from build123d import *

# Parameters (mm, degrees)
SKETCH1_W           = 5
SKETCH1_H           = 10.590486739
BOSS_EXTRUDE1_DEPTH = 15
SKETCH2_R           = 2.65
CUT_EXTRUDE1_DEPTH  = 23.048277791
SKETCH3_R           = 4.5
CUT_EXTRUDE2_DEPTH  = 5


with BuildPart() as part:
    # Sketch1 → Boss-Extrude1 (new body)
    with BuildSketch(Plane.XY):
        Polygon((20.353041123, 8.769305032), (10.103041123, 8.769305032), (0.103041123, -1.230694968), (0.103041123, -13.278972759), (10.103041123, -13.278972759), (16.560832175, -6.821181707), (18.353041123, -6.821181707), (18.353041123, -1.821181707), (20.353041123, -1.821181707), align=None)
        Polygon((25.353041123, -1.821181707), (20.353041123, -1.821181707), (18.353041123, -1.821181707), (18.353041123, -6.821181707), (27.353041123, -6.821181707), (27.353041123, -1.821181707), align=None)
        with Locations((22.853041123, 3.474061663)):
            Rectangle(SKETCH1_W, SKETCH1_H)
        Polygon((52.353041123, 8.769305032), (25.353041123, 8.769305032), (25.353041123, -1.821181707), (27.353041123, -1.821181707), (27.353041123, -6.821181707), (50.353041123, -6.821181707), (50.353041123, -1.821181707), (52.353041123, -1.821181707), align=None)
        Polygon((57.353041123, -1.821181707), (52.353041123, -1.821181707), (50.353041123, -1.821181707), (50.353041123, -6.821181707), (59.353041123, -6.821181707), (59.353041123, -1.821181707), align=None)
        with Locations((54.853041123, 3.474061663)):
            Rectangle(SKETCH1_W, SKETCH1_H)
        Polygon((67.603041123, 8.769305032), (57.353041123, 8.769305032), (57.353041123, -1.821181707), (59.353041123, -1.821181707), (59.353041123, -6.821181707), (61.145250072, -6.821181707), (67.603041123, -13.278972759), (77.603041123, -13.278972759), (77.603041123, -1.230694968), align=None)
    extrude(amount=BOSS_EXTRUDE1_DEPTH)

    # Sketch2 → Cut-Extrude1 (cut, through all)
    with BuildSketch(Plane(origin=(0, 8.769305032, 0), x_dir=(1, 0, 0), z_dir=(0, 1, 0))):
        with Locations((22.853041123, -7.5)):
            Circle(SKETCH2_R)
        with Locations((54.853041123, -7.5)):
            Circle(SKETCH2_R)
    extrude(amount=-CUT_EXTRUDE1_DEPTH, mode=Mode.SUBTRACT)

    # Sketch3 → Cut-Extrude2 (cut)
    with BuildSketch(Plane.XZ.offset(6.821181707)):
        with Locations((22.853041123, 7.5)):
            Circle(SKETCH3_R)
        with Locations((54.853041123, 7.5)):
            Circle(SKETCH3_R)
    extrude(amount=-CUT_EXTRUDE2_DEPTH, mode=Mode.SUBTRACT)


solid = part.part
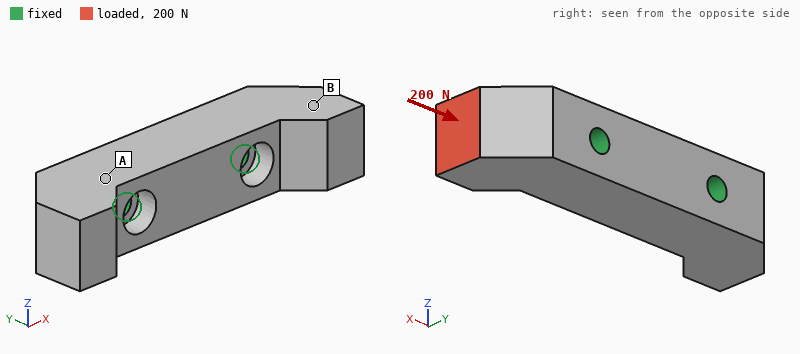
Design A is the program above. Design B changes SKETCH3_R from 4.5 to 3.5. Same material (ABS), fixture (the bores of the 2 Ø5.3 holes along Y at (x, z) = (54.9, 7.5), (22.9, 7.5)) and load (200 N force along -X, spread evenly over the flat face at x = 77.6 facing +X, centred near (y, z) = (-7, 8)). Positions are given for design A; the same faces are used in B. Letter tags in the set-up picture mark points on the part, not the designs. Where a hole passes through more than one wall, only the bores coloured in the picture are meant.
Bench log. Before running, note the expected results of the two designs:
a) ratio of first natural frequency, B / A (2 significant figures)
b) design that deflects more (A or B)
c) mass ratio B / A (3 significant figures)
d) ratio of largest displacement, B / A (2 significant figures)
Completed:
1.0
A
1.01
0.90
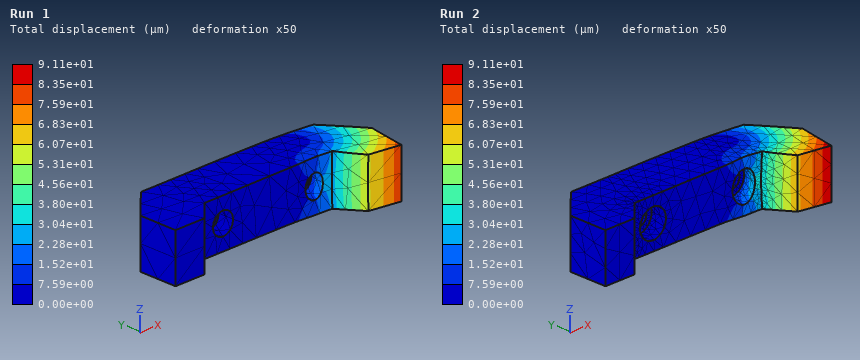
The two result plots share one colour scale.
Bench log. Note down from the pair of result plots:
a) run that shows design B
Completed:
Run 1
